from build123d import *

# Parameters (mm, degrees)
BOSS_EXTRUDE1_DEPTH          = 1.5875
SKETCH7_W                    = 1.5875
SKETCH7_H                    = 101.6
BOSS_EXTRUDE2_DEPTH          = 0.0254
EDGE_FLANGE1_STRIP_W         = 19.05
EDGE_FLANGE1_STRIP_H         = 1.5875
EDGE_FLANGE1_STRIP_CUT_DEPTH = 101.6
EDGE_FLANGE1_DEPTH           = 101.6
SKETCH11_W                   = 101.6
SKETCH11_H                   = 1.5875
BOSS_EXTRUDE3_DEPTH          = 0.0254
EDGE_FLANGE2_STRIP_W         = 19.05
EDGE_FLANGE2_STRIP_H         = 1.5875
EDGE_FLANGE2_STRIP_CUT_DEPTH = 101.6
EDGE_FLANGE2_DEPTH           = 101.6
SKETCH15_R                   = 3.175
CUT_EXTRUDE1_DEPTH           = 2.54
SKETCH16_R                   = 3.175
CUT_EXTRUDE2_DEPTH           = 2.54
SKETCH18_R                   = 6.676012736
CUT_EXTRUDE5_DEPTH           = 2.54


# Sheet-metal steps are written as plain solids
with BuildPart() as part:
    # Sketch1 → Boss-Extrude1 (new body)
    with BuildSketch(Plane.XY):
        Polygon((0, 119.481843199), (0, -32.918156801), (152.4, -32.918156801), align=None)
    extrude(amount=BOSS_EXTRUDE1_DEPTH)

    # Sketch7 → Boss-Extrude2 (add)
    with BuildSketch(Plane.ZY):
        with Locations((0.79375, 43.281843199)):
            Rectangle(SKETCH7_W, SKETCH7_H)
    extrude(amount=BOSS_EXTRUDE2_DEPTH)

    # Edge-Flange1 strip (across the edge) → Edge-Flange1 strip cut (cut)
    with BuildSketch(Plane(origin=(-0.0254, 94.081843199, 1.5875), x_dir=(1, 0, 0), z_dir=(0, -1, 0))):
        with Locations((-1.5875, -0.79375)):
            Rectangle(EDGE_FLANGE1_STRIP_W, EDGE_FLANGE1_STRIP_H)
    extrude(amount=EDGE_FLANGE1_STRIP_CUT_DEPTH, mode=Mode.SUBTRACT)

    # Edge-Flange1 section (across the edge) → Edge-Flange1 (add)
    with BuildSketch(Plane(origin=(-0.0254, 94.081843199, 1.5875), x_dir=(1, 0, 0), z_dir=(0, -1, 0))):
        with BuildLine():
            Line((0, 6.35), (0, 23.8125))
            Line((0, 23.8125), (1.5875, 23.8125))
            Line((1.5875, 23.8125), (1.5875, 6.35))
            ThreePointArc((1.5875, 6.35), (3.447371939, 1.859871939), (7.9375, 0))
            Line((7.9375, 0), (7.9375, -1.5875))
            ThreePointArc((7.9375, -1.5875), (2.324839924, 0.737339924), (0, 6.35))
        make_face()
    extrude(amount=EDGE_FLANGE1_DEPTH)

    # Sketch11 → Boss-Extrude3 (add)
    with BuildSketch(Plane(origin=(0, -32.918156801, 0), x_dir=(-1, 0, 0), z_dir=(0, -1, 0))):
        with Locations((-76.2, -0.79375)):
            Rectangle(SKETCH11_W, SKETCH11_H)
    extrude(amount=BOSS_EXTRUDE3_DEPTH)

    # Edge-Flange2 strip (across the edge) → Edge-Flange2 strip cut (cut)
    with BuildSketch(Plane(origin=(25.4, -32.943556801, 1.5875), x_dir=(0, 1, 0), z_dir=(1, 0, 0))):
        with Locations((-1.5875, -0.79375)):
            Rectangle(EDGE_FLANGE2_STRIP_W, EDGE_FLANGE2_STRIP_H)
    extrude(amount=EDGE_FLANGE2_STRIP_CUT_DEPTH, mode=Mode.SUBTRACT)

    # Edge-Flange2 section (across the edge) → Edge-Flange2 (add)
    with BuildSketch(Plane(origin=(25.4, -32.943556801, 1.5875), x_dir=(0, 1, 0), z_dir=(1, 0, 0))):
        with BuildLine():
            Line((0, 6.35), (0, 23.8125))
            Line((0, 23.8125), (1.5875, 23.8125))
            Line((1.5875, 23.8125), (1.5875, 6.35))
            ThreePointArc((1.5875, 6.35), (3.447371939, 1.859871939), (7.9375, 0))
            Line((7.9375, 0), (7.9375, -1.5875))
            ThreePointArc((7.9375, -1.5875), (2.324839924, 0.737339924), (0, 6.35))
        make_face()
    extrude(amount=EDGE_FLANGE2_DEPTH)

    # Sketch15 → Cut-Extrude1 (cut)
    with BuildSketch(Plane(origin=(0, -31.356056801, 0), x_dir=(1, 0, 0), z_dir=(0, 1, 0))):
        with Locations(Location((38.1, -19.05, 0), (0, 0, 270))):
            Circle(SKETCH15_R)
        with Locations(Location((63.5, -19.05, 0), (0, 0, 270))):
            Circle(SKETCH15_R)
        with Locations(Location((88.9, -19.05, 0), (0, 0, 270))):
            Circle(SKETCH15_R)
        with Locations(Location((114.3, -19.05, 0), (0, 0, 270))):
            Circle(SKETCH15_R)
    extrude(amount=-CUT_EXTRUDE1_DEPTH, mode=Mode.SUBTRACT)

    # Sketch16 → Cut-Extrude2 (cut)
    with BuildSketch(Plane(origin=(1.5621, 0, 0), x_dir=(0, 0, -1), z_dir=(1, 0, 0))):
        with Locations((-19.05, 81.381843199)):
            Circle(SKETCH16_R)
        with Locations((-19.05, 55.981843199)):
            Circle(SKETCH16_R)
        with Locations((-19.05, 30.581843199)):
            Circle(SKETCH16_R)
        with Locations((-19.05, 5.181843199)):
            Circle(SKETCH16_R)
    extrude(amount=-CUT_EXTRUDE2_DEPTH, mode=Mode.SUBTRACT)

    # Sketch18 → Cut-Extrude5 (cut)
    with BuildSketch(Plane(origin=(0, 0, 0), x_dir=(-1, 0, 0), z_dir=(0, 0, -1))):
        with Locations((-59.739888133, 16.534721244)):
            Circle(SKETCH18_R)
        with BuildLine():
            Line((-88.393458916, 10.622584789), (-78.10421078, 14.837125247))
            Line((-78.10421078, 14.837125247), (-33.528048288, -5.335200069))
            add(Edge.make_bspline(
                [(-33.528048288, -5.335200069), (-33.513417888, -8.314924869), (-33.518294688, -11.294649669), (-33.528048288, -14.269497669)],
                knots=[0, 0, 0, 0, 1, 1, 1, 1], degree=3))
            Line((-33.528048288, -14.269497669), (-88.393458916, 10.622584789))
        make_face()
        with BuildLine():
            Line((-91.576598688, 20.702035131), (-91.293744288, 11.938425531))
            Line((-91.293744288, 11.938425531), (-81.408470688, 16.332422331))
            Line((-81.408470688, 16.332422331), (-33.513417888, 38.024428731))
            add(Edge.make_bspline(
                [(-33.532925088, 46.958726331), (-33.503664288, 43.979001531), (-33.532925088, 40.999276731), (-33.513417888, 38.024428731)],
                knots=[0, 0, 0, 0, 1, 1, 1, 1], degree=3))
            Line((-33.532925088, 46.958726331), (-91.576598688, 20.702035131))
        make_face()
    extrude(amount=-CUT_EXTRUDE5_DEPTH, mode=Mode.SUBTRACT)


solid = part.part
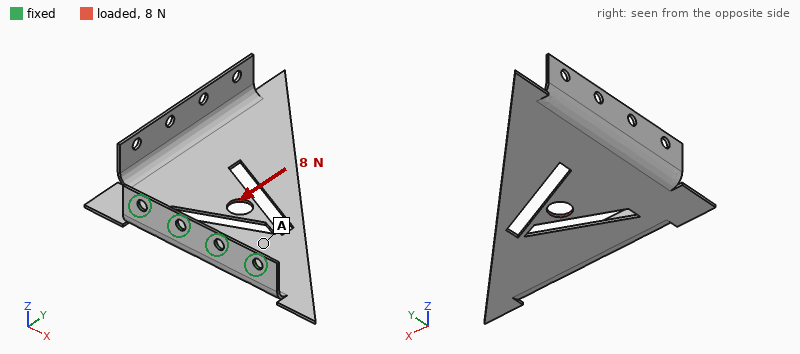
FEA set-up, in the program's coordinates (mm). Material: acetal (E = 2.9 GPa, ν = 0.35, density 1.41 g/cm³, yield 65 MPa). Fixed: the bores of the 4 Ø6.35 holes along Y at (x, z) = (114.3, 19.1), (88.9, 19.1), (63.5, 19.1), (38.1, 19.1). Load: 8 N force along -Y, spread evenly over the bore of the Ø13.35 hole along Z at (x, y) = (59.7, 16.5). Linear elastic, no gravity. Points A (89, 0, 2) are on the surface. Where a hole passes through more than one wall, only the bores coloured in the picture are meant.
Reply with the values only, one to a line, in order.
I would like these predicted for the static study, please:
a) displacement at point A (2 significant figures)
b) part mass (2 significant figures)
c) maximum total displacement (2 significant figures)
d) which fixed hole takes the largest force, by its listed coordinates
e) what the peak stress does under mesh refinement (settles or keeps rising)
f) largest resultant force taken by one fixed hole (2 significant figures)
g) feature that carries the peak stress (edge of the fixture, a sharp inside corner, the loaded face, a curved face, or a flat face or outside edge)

0.33 mm
32 g
2.2 mm
(38.1, 19.1)
keeps rising
3.6 N
edge of the fixture
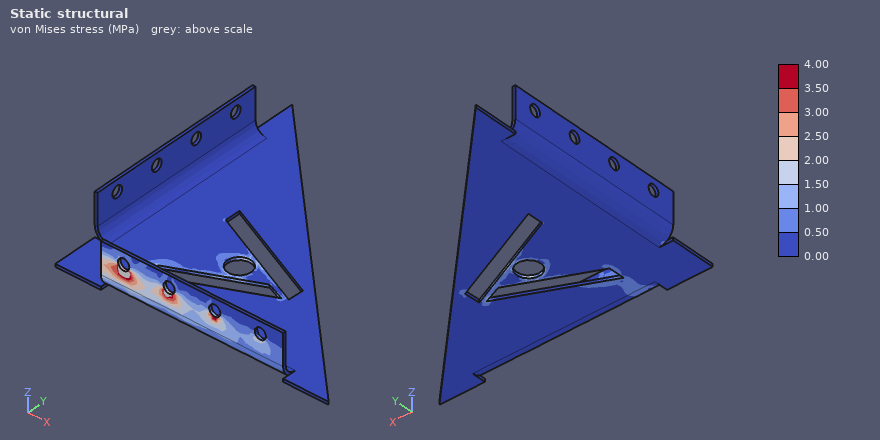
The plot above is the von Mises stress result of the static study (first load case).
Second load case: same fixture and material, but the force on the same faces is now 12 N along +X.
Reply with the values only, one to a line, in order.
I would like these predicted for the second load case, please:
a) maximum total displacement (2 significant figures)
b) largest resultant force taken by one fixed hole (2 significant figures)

2.4 mm
8.0 N
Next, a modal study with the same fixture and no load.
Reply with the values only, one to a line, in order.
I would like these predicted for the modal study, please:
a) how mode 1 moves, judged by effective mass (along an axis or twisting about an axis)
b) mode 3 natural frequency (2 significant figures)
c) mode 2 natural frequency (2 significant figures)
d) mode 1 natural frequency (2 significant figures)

along Z
110 Hz
79 Hz
16 Hz
